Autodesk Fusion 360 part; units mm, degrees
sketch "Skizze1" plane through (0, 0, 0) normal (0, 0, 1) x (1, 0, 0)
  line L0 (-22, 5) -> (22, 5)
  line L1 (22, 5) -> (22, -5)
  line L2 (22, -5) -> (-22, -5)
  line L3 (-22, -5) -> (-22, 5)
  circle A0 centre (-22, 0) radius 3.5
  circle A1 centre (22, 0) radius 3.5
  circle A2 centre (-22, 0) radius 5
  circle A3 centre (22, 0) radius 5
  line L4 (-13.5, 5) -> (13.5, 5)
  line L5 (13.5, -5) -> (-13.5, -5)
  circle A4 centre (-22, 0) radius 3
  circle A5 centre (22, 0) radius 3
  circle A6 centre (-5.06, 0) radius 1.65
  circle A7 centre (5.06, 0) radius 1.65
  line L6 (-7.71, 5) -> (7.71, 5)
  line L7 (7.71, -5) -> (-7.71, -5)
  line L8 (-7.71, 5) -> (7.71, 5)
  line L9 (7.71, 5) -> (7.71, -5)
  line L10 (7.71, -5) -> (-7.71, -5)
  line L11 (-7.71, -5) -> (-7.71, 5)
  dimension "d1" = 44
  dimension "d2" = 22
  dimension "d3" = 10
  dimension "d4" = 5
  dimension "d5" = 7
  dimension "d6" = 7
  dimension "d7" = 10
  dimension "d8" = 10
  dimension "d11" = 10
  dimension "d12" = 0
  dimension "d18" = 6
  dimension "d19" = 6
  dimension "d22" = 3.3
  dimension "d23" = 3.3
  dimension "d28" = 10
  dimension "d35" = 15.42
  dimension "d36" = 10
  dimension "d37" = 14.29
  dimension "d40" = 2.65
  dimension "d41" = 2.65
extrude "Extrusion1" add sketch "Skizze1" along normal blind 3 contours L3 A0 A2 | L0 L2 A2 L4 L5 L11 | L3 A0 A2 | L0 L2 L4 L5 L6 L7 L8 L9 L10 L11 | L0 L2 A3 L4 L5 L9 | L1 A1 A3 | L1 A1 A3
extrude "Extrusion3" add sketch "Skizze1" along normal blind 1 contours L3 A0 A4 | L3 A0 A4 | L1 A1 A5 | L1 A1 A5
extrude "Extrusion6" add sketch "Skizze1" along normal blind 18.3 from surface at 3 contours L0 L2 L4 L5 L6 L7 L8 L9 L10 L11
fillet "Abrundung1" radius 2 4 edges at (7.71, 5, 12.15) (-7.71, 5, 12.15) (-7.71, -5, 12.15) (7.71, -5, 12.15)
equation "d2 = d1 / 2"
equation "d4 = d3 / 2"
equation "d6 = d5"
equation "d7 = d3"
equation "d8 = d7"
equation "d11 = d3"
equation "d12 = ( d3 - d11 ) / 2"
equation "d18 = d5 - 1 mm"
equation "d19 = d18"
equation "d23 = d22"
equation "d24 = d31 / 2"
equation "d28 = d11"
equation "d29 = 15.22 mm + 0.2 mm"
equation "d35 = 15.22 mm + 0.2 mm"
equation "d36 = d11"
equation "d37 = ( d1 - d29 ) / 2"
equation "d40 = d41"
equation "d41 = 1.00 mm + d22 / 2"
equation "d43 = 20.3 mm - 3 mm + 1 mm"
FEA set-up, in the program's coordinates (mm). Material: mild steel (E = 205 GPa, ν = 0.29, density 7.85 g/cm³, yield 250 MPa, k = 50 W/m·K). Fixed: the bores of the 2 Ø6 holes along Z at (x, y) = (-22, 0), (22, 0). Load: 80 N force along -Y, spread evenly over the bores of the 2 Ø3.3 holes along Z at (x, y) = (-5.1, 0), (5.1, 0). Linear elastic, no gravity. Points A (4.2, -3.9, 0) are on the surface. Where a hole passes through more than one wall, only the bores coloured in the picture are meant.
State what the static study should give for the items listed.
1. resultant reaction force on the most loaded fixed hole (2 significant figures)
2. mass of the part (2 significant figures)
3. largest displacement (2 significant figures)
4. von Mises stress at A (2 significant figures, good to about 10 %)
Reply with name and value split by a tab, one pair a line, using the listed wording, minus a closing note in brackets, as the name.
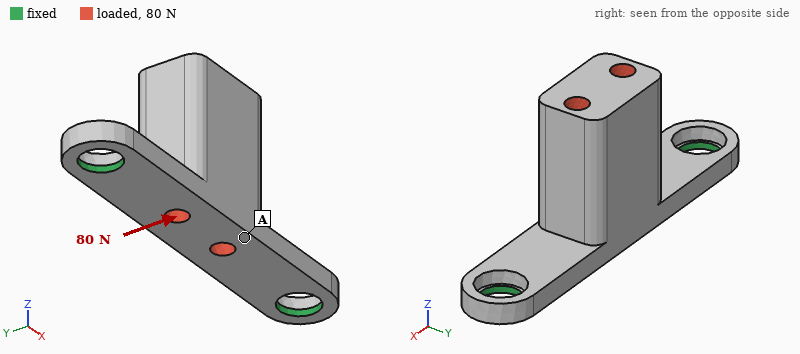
resultant reaction force on the most loaded fixed hole	40 N
mass of the part	29 g
largest displacement	21 µm
von Mises stress at A	8.1 MPa
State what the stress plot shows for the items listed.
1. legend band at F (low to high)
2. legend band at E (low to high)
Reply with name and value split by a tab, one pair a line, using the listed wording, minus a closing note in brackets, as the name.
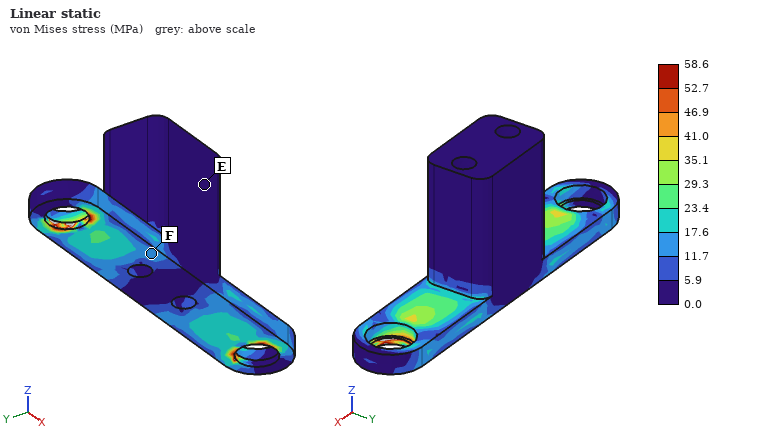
legend band at F	11.7 to 17.6 MPa
legend band at E	0.0 to 5.9 MPa
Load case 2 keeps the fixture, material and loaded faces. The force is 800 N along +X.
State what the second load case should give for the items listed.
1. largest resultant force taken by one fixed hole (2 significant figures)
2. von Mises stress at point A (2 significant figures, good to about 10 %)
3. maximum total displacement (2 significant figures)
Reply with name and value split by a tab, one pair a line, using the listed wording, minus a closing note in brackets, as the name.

largest resultant force taken by one fixed hole	470 N
von Mises stress at point A	30 MPa
maximum total displacement	30 µm
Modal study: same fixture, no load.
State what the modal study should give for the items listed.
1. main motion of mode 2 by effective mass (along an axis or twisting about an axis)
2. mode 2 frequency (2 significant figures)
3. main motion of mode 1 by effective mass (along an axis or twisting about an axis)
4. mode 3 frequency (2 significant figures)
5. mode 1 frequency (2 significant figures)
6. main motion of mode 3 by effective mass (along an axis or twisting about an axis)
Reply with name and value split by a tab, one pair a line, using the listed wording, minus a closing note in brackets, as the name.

main motion of mode 2 by effective mass	along Z
mode 2 frequency	5100 Hz
main motion of mode 1 by effective mass	along Y
mode 3 frequency	6300 Hz
mode 1 frequency	2500 Hz
main motion of mode 3 by effective mass	along X
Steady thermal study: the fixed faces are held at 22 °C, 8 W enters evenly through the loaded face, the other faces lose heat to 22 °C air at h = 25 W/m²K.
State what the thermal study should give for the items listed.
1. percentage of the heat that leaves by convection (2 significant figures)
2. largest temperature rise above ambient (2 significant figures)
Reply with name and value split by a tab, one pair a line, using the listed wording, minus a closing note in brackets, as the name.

percentage of the heat that leaves by convection	19 %
largest temperature rise above ambient	45 K
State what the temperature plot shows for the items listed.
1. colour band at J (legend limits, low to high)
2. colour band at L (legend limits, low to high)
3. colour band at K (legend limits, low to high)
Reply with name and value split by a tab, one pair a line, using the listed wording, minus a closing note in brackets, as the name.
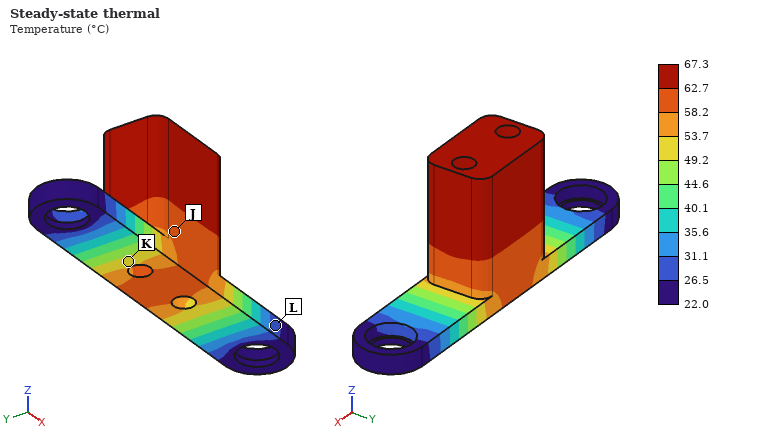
colour band at J	58.2 to 62.7 °C
colour band at L	26.5 to 31.1 °C
colour band at K	49.2 to 53.7 °C
